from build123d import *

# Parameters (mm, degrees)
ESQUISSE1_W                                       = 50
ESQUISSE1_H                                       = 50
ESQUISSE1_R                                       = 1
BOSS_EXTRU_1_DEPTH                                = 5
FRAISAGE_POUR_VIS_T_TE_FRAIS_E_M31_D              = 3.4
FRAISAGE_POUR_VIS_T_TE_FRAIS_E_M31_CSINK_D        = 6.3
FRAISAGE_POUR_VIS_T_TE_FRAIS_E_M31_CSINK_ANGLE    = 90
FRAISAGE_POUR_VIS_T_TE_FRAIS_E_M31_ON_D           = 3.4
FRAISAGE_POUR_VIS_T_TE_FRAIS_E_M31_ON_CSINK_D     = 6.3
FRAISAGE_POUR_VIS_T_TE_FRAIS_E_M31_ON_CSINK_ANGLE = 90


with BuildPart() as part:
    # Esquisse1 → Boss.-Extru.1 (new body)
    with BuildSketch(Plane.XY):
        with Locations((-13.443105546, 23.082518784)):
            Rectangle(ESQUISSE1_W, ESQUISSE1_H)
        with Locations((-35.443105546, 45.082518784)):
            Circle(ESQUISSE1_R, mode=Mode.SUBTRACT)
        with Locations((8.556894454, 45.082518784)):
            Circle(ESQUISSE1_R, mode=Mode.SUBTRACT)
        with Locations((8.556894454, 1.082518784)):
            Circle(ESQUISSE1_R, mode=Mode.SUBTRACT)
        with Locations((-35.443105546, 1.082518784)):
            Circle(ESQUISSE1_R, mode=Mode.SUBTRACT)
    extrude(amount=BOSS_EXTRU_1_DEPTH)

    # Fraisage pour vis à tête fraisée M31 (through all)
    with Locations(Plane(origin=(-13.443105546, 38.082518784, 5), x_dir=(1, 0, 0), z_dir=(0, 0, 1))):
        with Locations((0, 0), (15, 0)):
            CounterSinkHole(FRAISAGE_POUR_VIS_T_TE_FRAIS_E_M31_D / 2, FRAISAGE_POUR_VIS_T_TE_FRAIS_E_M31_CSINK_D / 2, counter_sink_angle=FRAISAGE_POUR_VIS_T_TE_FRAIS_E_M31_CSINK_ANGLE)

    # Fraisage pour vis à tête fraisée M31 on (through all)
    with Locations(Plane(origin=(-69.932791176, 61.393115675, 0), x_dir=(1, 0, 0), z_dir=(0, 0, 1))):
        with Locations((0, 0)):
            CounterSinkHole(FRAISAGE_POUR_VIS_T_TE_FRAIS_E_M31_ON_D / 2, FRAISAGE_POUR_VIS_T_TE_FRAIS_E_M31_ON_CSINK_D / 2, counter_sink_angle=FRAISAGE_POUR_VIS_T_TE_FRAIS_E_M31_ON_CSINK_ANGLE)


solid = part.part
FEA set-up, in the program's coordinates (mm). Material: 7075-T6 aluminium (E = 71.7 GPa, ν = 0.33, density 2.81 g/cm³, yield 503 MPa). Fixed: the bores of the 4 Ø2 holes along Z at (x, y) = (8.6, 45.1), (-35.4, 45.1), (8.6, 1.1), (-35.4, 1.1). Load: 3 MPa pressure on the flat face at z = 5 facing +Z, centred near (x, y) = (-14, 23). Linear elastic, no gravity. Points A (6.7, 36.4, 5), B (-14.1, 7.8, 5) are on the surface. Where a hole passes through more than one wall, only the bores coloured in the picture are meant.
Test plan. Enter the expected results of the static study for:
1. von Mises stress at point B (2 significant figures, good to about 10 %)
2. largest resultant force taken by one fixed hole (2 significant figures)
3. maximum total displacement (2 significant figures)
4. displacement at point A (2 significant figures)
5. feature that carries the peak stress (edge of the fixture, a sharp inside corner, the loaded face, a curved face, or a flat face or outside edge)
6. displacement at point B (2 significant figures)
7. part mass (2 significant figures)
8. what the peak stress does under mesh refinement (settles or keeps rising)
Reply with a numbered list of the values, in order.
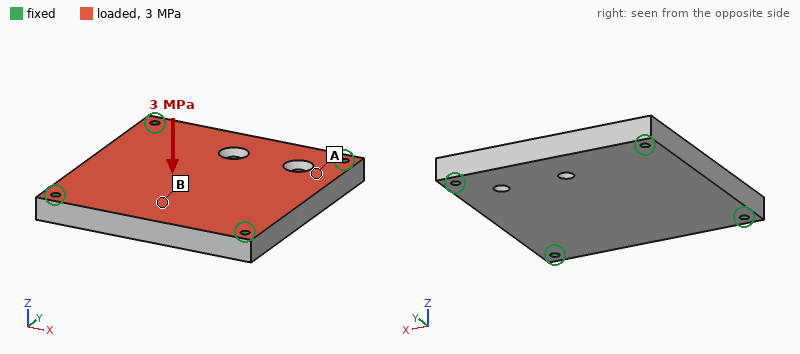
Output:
1. 79 MPa
2. 1.9 kN
3. 0.14 mm
4. 0.049 mm
5. edge of the fixture
6. 0.11 mm
7. 35 g
8. keeps rising
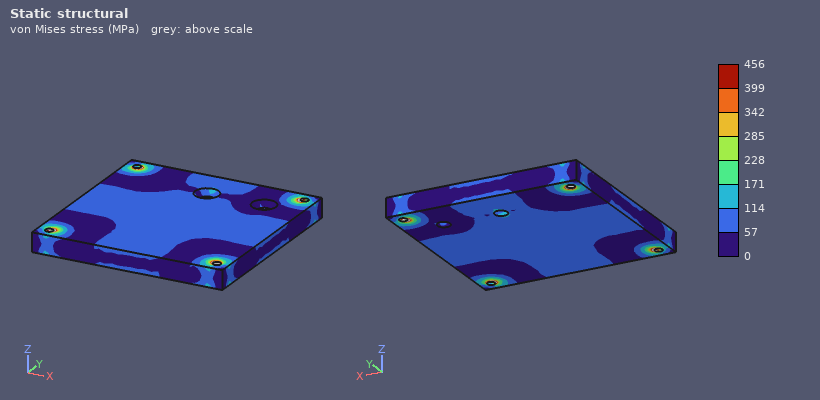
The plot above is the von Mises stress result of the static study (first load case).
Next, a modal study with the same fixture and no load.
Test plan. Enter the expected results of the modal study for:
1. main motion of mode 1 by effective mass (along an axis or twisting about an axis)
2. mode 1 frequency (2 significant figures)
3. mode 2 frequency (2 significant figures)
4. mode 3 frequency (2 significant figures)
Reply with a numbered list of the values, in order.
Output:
1. along Z
2. 7300 Hz
3. 13 kHz
4. 13 kHz
